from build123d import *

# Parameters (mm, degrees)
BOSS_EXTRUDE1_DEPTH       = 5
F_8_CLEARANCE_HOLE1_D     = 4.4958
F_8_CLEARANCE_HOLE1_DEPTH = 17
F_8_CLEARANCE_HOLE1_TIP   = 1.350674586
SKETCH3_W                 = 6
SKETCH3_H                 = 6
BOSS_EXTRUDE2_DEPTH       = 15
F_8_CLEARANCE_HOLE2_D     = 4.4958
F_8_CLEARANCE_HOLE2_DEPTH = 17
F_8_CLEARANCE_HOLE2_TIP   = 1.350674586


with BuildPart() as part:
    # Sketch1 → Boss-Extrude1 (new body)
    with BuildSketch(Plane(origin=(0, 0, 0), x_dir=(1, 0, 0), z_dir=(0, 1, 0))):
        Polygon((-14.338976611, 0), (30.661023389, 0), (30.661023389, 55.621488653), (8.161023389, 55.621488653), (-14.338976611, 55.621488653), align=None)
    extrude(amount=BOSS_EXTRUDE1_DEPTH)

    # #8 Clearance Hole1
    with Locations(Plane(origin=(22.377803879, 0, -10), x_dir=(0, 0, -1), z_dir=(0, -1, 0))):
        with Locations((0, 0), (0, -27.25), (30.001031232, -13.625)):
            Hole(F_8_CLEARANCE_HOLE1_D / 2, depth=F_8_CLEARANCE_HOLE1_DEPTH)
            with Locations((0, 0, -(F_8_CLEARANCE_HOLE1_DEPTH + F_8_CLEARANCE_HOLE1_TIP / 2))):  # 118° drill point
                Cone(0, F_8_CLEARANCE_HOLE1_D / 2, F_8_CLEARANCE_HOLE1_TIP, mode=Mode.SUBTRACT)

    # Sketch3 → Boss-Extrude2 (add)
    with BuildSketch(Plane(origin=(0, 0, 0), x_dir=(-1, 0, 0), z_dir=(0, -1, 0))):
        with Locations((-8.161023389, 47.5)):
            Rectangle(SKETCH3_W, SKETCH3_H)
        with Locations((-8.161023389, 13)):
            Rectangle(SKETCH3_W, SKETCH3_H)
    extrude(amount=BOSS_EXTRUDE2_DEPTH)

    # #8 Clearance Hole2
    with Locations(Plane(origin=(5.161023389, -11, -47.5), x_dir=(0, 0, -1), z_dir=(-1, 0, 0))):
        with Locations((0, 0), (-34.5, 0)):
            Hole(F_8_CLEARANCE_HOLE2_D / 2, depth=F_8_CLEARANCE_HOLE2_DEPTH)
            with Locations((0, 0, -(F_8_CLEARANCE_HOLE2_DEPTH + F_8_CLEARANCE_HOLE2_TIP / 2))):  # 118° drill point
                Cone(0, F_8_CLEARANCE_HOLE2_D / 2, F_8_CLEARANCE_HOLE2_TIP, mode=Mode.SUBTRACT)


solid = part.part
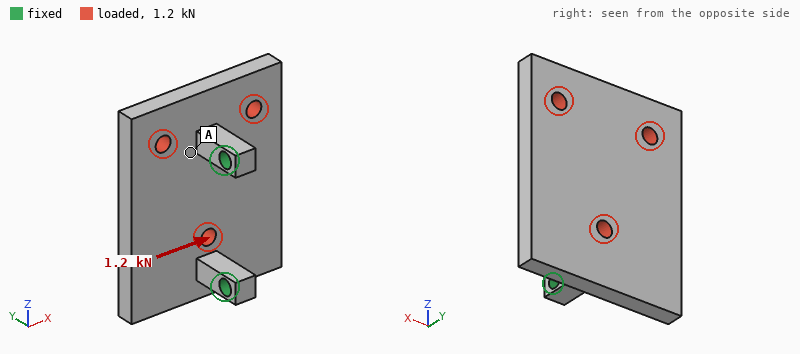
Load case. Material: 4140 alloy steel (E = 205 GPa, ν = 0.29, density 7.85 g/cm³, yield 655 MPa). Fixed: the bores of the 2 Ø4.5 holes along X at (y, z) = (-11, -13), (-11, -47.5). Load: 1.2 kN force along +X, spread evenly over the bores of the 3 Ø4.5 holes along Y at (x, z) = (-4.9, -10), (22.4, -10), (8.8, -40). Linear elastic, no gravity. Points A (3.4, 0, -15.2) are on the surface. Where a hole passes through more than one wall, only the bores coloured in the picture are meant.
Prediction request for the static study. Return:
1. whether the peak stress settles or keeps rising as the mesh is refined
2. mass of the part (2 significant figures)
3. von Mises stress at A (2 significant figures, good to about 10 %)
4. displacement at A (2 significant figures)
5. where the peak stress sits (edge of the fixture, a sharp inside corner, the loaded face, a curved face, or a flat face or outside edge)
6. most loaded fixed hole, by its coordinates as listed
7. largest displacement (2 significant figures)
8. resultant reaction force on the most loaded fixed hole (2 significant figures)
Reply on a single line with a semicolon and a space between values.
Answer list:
keeps rising; 100 g; 22 MPa; 19 µm; edge of the fixture; (-11, -13); 57 µm; 930 N
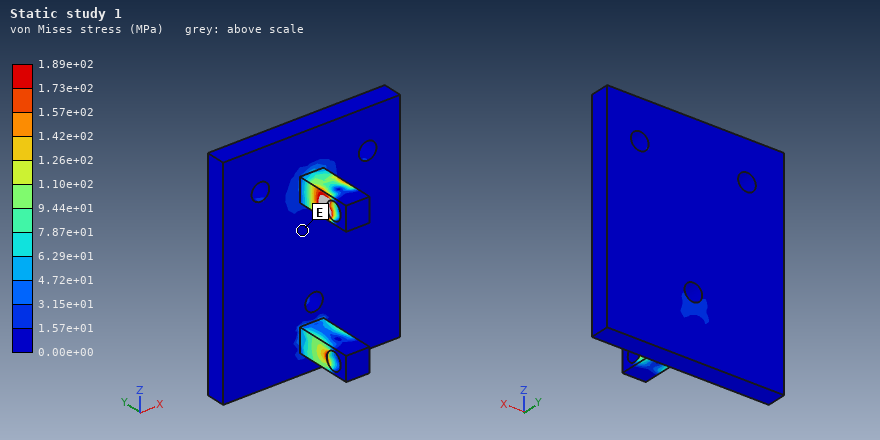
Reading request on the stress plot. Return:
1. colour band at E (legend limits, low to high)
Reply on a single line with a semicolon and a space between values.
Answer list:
0.00e+00 to 1.57e+01 MPa
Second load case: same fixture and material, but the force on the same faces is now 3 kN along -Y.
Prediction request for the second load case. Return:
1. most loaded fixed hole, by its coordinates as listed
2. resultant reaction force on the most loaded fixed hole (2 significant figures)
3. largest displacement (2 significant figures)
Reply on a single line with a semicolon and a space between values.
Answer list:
(-11, -13); 2.3 kN; 45 µm
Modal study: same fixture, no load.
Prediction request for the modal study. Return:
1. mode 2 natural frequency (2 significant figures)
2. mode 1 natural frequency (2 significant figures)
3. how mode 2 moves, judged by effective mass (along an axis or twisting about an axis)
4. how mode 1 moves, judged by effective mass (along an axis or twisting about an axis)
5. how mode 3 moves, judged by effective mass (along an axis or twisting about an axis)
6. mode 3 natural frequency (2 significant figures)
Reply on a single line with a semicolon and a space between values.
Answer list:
4900 Hz; 2200 Hz; twisting about Y; along X; along Z; 6200 Hz
